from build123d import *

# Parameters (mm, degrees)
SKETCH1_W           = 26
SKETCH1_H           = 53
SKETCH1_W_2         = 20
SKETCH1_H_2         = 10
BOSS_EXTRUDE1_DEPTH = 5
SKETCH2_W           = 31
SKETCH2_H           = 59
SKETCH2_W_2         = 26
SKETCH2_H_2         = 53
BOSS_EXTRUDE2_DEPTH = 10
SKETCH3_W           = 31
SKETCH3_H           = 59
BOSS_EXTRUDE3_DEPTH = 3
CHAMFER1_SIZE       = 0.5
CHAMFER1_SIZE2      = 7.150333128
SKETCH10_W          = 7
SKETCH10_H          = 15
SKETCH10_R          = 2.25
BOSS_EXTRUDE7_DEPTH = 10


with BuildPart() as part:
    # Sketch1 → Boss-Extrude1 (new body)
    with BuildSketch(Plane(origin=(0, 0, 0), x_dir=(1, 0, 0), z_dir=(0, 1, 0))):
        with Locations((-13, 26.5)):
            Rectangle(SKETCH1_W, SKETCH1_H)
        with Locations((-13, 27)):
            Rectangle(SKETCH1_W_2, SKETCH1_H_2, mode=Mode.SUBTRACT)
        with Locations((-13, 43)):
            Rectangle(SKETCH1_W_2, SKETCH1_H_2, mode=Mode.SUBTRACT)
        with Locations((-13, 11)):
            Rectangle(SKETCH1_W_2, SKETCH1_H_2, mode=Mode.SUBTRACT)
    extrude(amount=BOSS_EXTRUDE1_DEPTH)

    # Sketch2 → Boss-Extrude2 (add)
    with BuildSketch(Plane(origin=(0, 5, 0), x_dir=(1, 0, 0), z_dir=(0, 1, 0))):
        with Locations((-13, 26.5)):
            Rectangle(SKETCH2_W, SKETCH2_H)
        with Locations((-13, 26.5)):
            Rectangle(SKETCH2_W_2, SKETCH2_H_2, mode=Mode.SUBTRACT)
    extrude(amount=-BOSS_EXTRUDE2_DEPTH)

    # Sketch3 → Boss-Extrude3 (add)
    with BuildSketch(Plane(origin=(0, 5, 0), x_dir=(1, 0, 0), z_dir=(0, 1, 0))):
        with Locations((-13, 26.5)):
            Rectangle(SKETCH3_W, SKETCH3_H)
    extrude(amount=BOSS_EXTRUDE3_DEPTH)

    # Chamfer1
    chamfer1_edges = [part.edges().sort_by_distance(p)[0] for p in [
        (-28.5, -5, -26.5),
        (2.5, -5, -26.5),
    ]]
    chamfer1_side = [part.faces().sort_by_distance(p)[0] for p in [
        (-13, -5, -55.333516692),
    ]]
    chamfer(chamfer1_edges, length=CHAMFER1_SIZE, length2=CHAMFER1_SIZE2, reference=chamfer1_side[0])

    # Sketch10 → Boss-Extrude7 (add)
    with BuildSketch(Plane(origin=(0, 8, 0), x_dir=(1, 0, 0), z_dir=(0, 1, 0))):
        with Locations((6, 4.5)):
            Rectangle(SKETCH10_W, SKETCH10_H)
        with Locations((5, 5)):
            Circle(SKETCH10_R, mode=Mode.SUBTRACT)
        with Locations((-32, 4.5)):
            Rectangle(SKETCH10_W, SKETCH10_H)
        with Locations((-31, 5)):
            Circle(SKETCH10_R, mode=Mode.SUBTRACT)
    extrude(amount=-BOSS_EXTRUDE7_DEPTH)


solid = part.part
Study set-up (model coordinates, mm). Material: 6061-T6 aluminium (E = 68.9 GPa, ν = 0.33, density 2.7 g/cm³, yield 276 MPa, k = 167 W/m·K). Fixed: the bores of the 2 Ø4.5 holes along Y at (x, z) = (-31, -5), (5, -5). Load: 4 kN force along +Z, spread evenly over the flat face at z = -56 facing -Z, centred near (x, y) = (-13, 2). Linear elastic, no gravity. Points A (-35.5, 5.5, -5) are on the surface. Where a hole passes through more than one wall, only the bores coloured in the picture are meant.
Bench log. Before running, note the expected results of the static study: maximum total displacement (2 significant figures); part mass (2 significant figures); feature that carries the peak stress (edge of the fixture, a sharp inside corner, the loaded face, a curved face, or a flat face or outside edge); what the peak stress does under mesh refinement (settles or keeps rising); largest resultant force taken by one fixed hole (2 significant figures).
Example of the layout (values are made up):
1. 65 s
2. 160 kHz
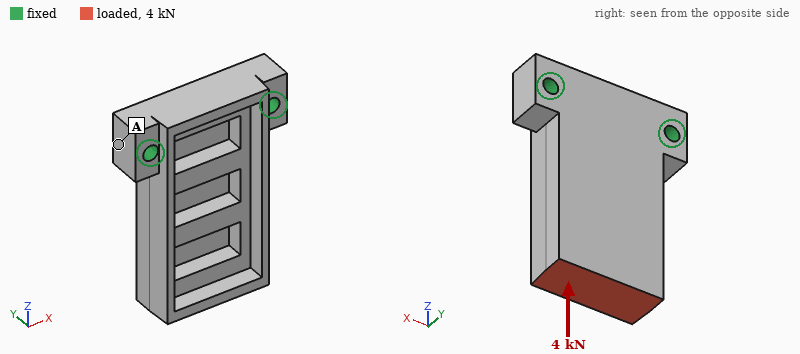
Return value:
1. 0.17 mm
2. 42 g
3. edge of the fixture
4. keeps rising
5. 2.0 kN
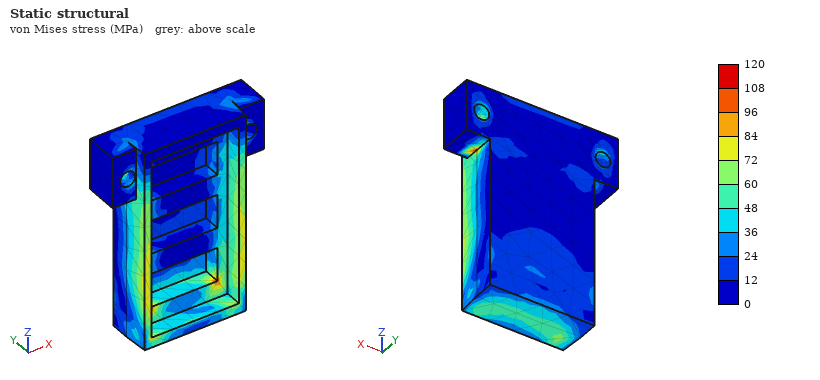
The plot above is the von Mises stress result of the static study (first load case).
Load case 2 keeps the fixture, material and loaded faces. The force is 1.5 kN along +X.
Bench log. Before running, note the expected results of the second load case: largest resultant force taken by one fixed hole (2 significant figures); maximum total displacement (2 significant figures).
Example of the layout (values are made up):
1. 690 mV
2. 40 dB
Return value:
1. 2.3 kN
2. 0.16 mm
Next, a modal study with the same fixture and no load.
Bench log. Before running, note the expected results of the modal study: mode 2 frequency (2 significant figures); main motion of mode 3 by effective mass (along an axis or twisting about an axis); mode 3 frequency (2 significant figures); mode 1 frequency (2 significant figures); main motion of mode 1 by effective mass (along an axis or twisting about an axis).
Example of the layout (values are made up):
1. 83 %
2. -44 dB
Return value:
1. 4900 Hz
2. along X
3. 7900 Hz
4. 2300 Hz
5. along Y
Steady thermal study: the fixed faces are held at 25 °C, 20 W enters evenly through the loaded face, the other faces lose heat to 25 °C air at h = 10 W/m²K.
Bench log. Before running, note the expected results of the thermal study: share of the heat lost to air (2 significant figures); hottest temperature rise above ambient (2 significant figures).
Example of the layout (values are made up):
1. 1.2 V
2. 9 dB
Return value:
1. 5.3 %
2. 35 K
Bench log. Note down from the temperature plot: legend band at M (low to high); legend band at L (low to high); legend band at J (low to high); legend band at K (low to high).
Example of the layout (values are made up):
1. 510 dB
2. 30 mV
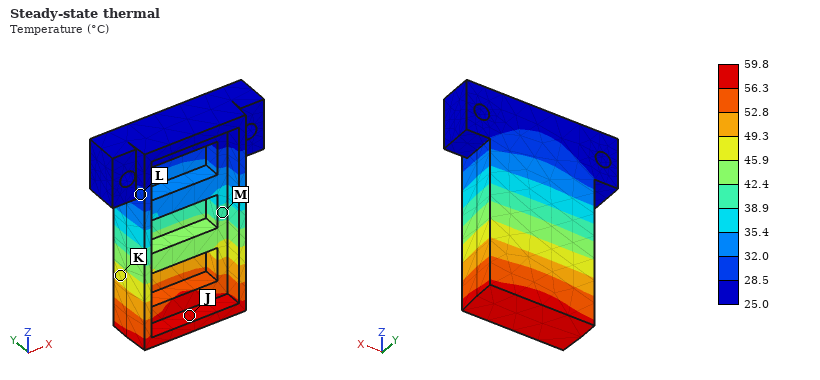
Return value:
1. 38.9 to 42.4 °C
2. 28.5 to 32.0 °C
3. 56.3 to 59.8 °C
4. 45.9 to 49.3 °C
